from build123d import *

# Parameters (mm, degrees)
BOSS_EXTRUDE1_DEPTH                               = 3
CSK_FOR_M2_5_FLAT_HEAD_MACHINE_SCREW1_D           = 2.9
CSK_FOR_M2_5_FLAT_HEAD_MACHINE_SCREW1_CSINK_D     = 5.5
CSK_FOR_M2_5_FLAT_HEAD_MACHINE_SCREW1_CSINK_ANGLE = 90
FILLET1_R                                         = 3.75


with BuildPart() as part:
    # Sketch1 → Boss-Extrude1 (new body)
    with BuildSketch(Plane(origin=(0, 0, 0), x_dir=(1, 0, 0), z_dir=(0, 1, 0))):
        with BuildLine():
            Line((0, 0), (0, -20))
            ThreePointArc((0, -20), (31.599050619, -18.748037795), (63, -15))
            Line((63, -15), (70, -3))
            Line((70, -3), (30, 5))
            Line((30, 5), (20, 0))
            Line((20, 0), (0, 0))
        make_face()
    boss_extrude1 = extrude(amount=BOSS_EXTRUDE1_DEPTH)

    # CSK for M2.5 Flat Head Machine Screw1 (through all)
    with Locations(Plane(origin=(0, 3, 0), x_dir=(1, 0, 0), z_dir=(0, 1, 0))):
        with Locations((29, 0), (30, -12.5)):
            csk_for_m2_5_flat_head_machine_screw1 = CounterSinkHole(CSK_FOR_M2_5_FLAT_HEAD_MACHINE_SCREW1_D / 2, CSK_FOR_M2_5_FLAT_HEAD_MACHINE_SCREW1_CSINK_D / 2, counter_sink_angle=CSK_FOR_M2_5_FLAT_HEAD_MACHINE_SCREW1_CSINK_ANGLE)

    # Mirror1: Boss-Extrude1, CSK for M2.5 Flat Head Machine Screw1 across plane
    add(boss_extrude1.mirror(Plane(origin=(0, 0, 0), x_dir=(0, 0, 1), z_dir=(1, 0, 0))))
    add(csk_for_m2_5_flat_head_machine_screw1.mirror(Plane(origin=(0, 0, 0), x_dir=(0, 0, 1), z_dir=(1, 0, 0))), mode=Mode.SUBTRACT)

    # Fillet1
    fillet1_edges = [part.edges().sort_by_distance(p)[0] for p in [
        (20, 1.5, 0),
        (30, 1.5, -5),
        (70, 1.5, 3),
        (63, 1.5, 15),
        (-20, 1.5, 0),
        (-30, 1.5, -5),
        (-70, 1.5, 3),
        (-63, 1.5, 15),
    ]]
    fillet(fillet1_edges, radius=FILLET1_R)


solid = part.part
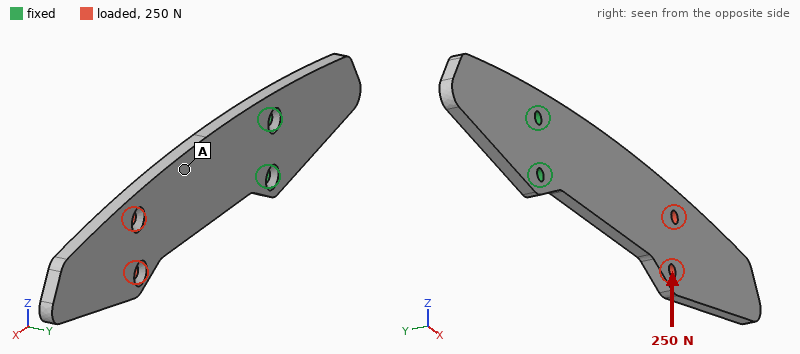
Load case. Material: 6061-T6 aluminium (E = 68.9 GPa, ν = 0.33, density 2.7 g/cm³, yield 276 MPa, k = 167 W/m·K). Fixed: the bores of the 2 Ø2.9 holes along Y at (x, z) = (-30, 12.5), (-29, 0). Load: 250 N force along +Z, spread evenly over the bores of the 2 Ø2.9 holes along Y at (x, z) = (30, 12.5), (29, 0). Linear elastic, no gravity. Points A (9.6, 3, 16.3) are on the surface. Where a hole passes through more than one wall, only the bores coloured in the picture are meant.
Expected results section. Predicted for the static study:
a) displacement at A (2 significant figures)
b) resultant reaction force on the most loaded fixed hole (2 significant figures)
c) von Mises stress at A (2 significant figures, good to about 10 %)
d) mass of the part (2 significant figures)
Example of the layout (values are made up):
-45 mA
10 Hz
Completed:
0.082 mm
1.1 kN
16 MPa
20 g
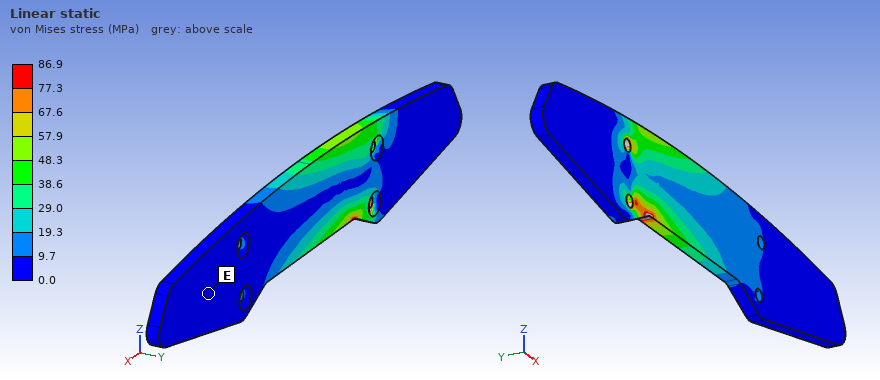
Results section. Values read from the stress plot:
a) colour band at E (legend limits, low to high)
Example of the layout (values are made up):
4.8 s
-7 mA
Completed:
0.0 to 9.7 MPa
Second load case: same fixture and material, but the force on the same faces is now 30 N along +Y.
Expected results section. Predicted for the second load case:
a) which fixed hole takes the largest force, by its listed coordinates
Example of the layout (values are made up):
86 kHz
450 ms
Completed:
(-29, 0)
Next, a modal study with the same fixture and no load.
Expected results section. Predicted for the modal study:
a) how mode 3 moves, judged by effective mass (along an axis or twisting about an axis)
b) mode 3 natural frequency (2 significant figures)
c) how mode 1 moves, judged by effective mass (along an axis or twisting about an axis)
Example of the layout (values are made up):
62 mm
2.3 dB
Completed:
along Z
1800 Hz
along Y
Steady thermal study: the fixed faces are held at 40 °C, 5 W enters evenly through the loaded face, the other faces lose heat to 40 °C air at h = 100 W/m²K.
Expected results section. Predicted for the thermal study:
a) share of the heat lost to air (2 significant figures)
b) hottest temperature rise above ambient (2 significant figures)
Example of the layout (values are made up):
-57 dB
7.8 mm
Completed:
68 %
14 K
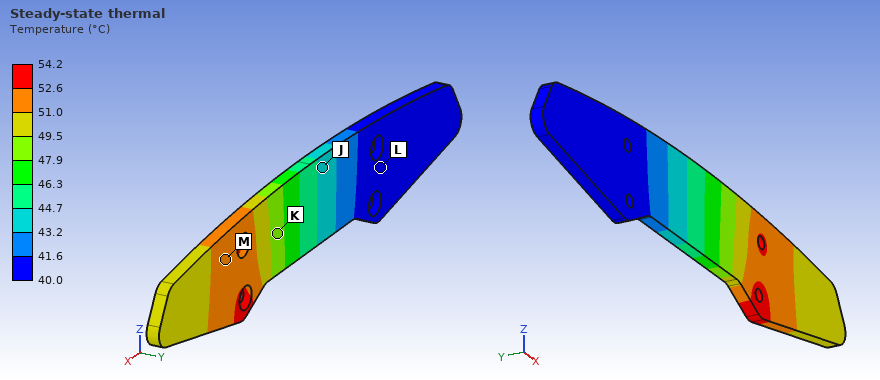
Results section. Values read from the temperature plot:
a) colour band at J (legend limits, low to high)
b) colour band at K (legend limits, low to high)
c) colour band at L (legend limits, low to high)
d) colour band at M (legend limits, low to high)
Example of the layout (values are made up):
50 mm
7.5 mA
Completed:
43.2 to 44.7 °C
47.9 to 49.5 °C
40.0 to 41.6 °C
51.0 to 52.6 °C
